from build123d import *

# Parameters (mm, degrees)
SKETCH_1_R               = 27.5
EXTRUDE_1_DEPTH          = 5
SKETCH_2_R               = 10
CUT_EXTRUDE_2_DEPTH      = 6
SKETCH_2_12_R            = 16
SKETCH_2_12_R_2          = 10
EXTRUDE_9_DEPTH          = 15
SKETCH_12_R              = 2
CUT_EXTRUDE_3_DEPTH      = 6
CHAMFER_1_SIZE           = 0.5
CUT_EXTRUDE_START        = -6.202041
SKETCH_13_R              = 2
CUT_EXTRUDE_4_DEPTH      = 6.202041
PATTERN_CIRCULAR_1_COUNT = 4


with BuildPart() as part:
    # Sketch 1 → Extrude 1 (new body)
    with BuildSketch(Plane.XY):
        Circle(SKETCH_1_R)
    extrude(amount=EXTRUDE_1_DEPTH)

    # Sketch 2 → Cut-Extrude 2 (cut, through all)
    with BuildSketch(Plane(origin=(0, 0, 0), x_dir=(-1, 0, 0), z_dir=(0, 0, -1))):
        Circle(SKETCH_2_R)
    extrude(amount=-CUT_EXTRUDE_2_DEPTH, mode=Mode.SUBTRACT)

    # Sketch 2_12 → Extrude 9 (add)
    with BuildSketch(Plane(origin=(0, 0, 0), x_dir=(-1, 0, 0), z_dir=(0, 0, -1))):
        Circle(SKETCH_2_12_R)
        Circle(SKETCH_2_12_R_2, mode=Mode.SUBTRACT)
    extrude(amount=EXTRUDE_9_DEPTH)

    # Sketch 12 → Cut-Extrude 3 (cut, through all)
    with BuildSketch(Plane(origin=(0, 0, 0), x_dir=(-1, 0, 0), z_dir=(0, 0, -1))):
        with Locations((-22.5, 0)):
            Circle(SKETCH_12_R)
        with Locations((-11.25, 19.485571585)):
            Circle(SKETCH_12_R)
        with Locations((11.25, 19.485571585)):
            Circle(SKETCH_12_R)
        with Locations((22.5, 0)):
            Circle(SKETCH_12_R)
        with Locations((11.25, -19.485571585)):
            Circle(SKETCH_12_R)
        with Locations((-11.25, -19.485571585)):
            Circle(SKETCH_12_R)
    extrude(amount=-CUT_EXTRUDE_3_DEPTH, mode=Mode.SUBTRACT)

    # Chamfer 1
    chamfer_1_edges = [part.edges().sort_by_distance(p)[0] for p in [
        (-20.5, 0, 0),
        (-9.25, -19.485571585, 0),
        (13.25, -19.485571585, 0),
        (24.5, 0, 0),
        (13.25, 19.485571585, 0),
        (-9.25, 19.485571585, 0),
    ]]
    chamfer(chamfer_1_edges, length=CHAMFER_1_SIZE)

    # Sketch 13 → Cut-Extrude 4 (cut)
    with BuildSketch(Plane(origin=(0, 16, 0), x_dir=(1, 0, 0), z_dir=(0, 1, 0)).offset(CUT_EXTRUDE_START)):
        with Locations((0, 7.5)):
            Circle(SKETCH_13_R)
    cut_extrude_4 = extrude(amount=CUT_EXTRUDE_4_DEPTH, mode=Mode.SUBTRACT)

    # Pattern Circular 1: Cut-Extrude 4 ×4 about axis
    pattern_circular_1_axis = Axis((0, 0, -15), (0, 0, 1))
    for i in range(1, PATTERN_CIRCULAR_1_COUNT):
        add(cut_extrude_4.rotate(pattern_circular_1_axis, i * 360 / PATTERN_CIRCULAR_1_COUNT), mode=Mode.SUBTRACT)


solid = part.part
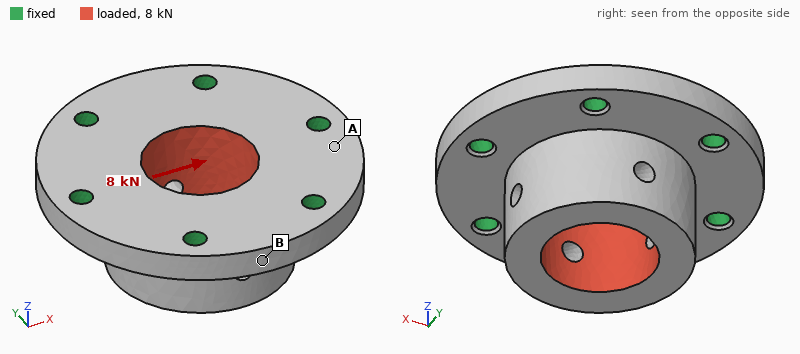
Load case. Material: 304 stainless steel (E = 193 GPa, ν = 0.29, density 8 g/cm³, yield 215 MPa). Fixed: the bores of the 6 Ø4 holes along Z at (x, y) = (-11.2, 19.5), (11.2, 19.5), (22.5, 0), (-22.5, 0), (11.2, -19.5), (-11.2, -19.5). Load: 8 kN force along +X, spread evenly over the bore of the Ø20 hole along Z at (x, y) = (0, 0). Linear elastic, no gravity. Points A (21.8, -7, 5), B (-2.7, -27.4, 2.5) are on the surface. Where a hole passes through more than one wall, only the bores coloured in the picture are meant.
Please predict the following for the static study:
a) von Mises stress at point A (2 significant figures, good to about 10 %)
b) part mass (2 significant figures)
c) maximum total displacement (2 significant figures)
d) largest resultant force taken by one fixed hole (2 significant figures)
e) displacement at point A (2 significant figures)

16 MPa
140 g
8.0 µm
2.1 kN
1.4 µm
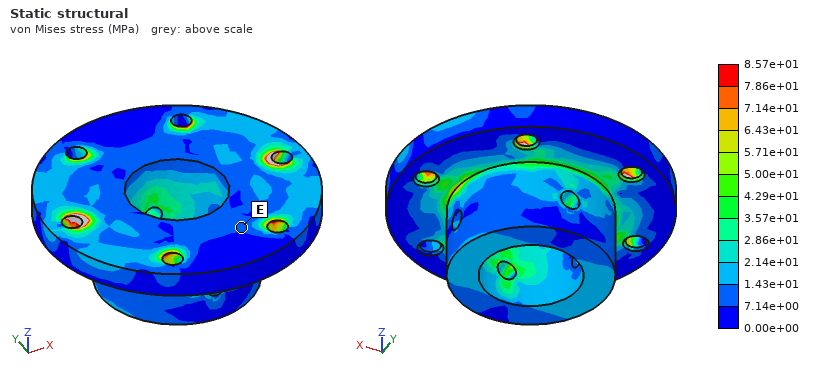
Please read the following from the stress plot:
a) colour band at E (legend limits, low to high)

7.14e+00 to 1.43e+01 MPa
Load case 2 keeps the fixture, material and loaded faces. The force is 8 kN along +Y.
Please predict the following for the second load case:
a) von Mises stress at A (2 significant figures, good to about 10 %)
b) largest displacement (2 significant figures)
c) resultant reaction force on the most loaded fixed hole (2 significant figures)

9.8 MPa
8.0 µm
1.8 kN
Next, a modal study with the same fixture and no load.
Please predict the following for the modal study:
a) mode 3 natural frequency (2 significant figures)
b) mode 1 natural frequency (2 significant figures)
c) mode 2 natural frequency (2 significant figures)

21 kHz
20 kHz
20 kHz
